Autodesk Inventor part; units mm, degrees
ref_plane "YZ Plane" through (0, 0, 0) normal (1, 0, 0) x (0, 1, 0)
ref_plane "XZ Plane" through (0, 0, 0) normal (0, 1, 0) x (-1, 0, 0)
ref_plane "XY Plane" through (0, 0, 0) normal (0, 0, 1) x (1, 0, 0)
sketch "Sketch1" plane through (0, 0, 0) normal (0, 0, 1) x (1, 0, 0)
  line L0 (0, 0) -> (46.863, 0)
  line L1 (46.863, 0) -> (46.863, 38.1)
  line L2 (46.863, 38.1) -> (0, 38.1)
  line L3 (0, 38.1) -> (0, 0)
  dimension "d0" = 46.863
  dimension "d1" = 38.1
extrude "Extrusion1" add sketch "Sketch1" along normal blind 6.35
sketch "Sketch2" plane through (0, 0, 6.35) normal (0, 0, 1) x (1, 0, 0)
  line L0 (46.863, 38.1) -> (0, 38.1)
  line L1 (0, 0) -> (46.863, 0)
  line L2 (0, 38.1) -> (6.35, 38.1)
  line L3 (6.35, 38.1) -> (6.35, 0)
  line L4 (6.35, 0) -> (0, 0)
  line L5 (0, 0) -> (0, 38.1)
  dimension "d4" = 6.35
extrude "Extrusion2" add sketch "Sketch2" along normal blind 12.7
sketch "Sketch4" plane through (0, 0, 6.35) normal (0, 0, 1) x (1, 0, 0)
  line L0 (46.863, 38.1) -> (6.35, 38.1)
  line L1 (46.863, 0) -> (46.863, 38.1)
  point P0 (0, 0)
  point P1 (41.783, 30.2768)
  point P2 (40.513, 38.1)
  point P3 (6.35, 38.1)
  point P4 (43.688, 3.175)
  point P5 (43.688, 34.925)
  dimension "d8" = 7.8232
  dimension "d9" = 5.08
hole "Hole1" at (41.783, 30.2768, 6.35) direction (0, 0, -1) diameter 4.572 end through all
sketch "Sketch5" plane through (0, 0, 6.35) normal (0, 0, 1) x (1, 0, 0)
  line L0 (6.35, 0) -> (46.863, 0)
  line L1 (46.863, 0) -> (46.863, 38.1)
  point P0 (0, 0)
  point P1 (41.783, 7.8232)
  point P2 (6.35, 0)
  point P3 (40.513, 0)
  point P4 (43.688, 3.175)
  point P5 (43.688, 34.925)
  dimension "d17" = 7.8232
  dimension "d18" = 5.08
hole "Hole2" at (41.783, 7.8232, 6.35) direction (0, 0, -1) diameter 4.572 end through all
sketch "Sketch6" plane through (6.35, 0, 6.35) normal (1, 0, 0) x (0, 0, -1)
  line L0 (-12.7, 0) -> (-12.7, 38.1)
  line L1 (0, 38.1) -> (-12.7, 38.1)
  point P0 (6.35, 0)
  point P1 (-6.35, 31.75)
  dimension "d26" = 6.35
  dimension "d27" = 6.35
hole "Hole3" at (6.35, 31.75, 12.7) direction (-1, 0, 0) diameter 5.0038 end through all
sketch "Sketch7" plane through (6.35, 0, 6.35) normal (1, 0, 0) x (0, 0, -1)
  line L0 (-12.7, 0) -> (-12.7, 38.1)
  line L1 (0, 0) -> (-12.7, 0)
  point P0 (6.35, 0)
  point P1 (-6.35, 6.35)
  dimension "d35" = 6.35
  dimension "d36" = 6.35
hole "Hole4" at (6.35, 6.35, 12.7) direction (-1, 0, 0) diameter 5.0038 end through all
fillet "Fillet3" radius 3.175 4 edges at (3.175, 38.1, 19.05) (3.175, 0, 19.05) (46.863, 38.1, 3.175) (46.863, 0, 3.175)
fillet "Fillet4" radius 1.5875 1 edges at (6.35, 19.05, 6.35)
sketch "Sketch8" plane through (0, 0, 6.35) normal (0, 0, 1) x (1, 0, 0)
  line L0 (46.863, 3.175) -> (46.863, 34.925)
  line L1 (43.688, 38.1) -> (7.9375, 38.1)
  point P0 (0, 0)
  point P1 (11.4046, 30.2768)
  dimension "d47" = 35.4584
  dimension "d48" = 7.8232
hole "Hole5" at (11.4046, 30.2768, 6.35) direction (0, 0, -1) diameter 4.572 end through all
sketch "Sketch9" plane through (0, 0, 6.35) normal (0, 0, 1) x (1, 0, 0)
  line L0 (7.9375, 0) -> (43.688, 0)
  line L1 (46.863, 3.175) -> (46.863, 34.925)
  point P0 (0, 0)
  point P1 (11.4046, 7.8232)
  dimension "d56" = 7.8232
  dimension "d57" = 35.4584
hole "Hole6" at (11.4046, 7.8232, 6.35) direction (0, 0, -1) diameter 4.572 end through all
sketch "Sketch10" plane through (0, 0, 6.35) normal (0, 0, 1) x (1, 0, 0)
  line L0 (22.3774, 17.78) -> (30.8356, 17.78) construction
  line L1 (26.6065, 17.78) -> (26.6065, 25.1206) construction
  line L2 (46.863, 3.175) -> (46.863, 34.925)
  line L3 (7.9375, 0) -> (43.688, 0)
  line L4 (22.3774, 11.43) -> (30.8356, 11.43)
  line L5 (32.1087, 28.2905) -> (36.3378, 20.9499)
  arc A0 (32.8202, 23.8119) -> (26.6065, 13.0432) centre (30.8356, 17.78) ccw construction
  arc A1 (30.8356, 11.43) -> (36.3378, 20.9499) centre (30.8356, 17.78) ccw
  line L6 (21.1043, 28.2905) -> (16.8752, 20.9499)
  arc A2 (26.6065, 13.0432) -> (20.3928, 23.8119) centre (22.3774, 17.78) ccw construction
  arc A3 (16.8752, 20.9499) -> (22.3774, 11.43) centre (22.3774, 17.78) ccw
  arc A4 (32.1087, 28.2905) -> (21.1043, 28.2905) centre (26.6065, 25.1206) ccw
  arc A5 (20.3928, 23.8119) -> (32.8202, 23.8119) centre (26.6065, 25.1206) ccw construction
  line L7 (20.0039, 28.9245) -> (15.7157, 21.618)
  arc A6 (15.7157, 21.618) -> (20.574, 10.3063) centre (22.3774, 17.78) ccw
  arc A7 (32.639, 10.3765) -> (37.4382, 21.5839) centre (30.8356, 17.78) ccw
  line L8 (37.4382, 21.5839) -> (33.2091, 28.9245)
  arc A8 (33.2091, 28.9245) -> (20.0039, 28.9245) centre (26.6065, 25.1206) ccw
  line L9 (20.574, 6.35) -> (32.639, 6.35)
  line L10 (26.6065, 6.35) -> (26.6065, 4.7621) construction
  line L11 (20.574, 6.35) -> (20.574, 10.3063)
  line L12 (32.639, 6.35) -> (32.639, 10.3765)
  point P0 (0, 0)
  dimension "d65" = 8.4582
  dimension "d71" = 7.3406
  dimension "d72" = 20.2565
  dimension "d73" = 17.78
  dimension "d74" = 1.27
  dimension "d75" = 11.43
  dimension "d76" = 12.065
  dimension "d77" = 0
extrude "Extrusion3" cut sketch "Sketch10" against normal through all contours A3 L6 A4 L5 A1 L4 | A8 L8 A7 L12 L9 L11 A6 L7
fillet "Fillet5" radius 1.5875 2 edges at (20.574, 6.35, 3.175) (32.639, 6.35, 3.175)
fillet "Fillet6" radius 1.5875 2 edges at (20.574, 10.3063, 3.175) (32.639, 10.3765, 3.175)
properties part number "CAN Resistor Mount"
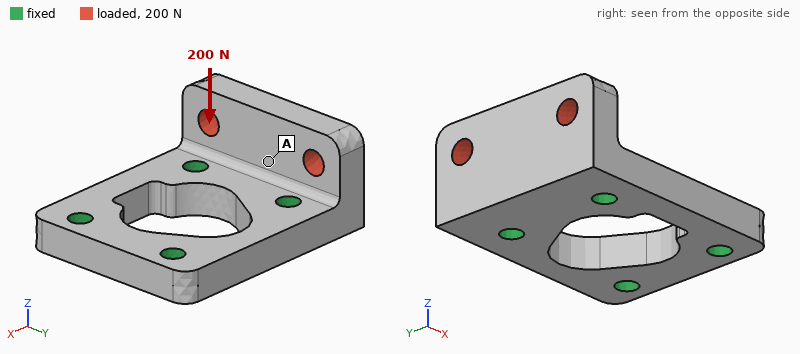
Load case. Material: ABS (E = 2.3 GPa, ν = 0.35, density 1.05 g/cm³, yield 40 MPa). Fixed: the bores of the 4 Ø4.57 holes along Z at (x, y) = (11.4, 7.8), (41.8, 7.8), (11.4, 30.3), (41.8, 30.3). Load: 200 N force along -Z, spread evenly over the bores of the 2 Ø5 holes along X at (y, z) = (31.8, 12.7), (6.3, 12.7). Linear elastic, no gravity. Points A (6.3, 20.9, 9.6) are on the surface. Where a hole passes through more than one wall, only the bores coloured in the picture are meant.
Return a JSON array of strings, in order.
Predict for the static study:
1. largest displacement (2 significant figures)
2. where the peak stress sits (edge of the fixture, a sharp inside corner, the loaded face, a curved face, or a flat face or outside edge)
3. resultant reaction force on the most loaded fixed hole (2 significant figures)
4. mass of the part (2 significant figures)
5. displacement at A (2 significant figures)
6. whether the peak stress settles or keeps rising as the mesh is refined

["79 µm", "edge of the fixture", "100 N", "11 g", "29 µm", "keeps rising"]
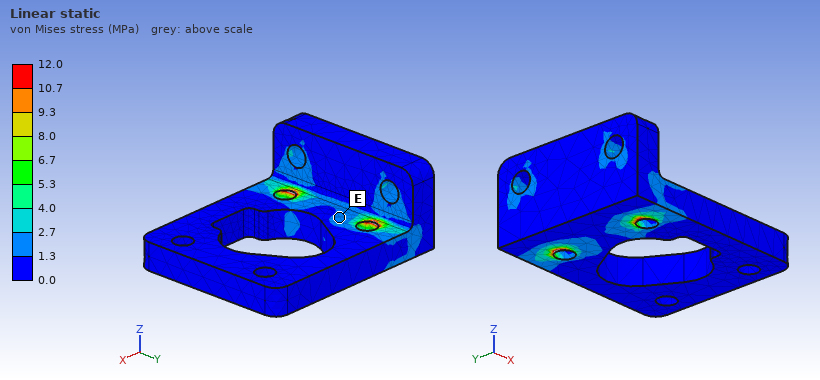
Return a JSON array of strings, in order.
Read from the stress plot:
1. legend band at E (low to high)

["1.3 to 2.7 MPa"]
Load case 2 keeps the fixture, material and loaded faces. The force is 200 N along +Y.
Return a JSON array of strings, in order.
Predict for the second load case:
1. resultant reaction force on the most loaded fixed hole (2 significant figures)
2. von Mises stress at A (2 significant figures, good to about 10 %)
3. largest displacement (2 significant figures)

["130 N", "2.5 MPa", "45 µm"]
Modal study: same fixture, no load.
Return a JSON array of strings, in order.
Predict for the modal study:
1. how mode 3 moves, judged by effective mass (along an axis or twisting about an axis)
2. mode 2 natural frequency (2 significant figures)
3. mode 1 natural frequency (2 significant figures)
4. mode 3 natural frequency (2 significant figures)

["along Y", "5400 Hz", "3500 Hz", "7800 Hz"]
